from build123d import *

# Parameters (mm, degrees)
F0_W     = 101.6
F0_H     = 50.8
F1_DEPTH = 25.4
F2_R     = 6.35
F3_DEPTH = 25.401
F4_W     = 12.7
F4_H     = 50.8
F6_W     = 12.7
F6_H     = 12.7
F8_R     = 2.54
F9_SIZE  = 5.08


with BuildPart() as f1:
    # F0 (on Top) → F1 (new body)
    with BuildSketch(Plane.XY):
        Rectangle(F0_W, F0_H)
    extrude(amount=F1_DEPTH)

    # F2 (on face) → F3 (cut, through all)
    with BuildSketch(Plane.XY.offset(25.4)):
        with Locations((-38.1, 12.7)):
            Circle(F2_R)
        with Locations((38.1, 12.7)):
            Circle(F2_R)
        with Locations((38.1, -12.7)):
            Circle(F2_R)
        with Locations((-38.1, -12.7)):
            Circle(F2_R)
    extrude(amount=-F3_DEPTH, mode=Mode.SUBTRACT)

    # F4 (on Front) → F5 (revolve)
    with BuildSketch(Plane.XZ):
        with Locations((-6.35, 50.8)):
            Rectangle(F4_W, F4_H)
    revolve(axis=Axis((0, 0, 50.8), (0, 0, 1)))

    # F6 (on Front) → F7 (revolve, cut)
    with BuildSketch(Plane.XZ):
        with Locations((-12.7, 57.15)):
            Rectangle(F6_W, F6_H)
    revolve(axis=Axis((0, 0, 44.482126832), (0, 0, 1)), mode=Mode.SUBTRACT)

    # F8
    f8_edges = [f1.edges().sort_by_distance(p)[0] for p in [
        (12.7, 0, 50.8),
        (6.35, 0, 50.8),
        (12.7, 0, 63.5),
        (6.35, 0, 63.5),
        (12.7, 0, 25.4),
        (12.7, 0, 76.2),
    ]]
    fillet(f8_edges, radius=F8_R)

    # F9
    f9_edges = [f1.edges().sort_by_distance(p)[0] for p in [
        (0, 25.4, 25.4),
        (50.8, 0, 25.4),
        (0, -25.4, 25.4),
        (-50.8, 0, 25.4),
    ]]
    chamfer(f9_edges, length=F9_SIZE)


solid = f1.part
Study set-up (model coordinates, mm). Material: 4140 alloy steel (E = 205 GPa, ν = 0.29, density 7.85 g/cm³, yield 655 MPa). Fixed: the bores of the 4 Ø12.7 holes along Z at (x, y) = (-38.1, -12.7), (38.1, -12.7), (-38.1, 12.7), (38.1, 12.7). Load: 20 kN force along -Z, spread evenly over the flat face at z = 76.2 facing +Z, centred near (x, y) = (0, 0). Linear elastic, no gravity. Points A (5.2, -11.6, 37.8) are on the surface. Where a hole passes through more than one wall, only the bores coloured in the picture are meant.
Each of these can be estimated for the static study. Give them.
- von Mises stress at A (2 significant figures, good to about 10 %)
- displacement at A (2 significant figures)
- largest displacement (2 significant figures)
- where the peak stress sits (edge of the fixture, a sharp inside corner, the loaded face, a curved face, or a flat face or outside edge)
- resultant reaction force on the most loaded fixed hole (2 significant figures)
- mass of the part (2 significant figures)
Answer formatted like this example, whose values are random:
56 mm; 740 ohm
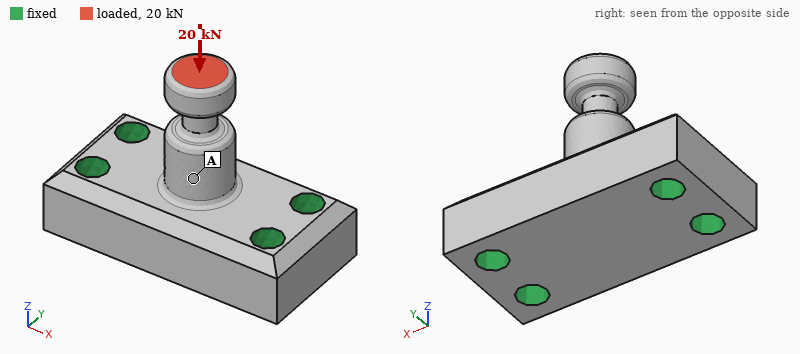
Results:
34 MPa; 7.8 µm; 26 µm; a curved face; 5.1 kN; 1.1 kg
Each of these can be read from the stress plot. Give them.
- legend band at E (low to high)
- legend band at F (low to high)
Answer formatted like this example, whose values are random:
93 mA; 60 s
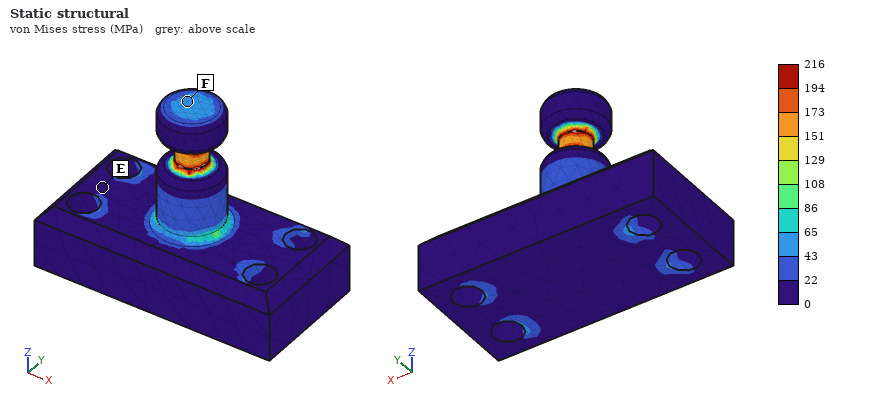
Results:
0 to 22 MPa; 43 to 65 MPa
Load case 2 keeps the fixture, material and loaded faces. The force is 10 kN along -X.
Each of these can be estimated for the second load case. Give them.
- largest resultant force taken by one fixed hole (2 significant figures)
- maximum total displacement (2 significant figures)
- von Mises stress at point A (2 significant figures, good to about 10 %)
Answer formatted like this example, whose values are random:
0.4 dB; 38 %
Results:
6.3 kN; 0.39 mm; 99 MPa
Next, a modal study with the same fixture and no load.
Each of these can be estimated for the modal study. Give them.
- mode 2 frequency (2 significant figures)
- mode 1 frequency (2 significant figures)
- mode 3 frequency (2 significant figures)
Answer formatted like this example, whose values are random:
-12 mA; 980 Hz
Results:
4500 Hz; 4300 Hz; 9100 Hz
